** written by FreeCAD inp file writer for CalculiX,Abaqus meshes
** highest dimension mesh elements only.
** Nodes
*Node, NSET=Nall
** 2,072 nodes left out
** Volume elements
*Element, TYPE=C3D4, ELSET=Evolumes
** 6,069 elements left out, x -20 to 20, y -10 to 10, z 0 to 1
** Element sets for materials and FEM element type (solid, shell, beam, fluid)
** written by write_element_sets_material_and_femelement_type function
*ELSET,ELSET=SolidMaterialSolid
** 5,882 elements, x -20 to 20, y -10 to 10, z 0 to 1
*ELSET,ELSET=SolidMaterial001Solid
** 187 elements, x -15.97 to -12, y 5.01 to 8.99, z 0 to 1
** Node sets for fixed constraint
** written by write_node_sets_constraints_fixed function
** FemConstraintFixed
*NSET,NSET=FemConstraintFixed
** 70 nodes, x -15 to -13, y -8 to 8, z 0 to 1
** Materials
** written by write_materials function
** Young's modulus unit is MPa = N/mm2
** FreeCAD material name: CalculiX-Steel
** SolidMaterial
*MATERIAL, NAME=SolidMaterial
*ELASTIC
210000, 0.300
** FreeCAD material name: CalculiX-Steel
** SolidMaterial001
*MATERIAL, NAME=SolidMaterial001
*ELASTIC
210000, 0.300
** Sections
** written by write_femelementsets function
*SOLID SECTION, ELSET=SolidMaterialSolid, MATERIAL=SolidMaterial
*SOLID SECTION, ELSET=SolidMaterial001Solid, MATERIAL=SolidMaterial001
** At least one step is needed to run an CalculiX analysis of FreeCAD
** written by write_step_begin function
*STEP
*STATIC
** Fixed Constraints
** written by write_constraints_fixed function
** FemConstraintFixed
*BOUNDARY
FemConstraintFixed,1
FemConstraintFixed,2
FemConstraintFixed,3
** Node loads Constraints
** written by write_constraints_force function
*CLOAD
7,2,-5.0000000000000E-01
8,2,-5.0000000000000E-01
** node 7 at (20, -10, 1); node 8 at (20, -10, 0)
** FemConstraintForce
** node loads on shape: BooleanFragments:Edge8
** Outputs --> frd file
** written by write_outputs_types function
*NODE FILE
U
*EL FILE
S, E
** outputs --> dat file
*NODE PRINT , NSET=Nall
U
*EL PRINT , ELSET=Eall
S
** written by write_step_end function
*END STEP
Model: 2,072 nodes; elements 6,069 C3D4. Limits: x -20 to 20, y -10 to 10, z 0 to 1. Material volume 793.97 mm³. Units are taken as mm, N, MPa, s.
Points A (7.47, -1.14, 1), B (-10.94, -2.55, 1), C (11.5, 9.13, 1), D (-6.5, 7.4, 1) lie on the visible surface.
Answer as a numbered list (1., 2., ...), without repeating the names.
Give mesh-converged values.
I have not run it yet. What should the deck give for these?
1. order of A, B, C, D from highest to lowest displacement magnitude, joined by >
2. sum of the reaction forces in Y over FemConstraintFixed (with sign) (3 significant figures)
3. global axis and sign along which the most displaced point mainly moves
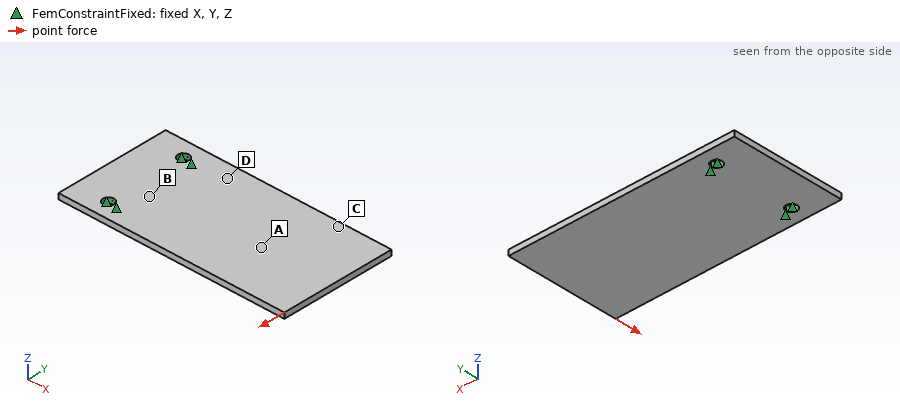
1. C > A > D > B
2. 1.00 N
3. -Y
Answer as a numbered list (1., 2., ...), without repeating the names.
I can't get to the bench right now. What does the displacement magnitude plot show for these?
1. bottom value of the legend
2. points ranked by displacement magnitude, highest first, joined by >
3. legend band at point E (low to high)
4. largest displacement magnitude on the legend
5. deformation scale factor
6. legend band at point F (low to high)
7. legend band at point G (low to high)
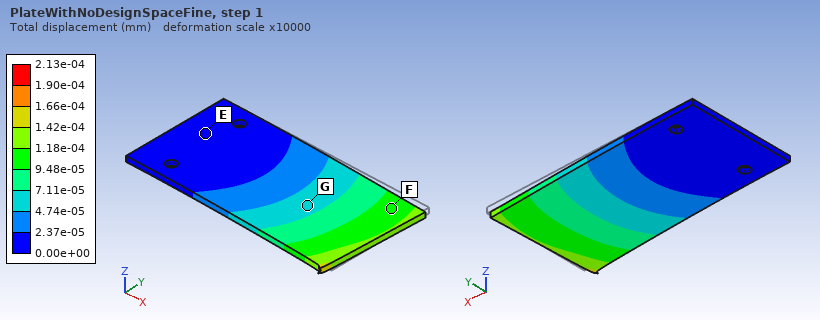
1. 0.00e+00 mm
2. F > G > E
3. 0.00e+00 to 2.37e-05 mm
4. 2.13e-04 mm
5. 10000
6. 9.48e-05 to 1.18e-04 mm
7. 4.74e-05 to 7.11e-05 mm
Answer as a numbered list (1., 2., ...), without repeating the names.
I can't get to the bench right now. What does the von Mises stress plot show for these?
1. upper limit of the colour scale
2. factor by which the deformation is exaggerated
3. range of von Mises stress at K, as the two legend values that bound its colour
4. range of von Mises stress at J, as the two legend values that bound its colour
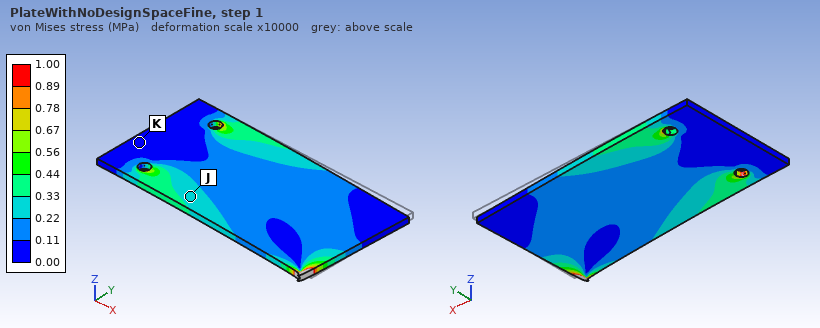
1. 1.00 MPa
2. 10000
3. 0.00 to 0.11 MPa
4. 0.22 to 0.33 MPa
